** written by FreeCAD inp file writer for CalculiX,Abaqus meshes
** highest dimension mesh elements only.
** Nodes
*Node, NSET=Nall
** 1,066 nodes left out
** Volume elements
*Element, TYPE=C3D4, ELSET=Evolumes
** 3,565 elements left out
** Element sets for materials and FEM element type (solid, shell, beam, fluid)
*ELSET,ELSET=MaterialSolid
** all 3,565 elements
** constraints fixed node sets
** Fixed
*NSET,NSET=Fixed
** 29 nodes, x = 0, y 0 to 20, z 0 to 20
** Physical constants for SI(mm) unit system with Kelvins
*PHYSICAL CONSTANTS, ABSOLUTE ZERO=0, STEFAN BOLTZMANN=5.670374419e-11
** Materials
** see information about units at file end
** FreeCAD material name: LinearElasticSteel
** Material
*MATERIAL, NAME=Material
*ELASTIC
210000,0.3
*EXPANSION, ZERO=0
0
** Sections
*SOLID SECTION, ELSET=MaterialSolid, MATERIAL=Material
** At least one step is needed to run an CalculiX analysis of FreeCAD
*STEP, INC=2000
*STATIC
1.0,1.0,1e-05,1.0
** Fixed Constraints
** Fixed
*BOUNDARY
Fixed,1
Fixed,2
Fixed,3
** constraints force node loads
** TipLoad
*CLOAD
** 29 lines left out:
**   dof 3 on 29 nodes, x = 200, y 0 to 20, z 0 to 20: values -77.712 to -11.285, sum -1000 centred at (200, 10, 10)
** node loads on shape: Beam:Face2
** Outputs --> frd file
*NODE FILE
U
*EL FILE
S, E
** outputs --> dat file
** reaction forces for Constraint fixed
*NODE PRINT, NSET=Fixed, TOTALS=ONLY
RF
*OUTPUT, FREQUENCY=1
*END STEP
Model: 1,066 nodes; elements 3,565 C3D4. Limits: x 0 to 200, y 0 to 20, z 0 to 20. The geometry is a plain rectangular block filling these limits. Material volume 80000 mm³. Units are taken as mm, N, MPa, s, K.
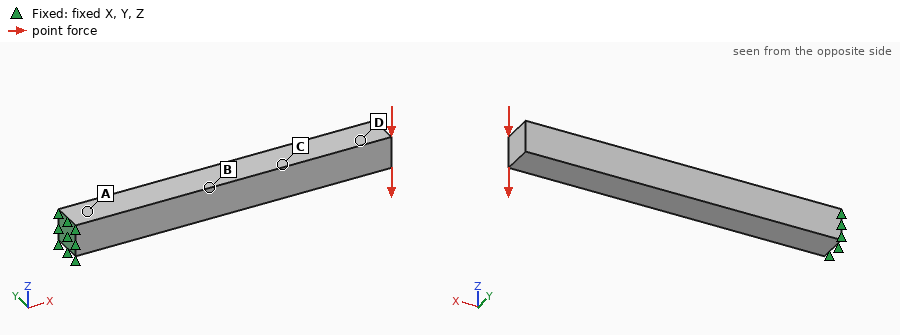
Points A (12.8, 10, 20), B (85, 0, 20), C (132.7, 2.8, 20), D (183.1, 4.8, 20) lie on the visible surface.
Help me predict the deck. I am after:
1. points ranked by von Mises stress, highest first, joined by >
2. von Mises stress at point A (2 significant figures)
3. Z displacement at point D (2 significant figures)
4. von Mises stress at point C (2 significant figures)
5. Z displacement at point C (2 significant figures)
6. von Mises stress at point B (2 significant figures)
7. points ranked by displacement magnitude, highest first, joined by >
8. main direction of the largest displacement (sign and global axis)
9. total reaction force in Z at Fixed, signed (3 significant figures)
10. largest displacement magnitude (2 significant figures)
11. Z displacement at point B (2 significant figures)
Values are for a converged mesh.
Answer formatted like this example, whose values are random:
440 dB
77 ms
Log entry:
A > B > C > D
140 MPa
-0.83 mm
50 MPa
-0.49 mm
86 MPa
D > C > B > A
-Z
1000 N
0.96 mm
-0.22 mm
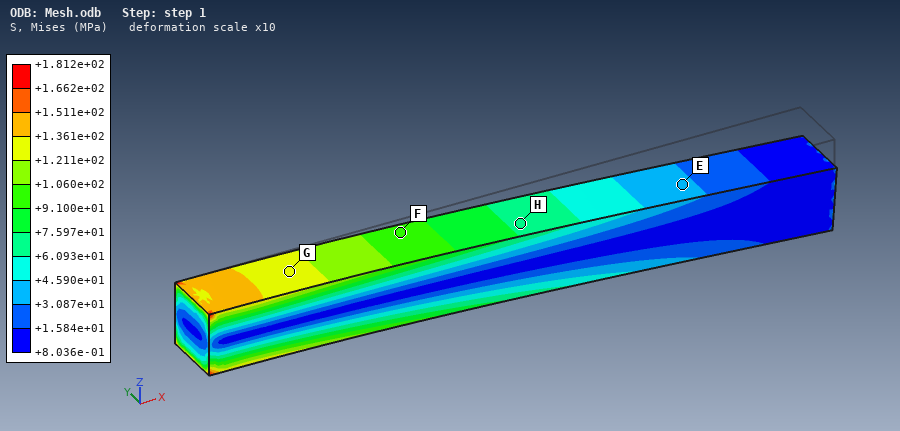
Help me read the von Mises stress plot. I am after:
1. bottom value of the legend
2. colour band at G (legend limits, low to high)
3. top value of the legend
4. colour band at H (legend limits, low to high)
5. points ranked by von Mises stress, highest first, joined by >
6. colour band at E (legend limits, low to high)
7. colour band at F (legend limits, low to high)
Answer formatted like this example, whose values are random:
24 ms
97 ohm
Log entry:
+8.036e-01 MPa
+1.211e+02 to +1.361e+02 MPa
+1.812e+02 MPa
+6.093e+01 to +7.597e+01 MPa
G > F > H > E
+3.087e+01 to +4.590e+01 MPa
+9.100e+01 to +1.060e+02 MPa
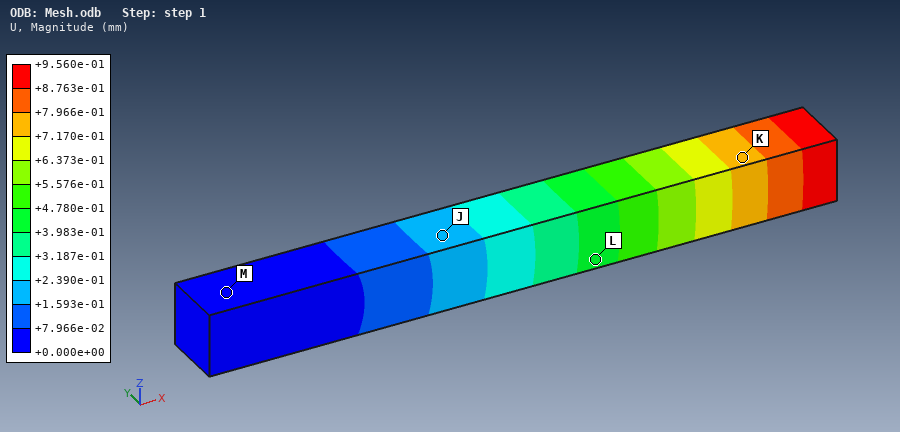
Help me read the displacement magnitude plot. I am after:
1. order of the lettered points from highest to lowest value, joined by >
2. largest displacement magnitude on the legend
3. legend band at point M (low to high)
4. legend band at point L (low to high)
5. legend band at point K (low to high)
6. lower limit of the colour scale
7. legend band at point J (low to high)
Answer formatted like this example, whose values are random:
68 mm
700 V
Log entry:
K > L > J > M
+9.560e-01 mm
+0.000e+00 to +7.966e-02 mm
+3.983e-01 to +4.780e-01 mm
+7.170e-01 to +7.966e-01 mm
+0.000e+00 mm
+1.593e-01 to +2.390e-01 mm
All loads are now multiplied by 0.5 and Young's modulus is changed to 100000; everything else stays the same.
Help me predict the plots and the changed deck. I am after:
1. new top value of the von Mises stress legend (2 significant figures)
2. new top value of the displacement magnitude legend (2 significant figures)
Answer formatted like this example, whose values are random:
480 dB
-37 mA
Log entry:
91 MPa
1.0 mm
